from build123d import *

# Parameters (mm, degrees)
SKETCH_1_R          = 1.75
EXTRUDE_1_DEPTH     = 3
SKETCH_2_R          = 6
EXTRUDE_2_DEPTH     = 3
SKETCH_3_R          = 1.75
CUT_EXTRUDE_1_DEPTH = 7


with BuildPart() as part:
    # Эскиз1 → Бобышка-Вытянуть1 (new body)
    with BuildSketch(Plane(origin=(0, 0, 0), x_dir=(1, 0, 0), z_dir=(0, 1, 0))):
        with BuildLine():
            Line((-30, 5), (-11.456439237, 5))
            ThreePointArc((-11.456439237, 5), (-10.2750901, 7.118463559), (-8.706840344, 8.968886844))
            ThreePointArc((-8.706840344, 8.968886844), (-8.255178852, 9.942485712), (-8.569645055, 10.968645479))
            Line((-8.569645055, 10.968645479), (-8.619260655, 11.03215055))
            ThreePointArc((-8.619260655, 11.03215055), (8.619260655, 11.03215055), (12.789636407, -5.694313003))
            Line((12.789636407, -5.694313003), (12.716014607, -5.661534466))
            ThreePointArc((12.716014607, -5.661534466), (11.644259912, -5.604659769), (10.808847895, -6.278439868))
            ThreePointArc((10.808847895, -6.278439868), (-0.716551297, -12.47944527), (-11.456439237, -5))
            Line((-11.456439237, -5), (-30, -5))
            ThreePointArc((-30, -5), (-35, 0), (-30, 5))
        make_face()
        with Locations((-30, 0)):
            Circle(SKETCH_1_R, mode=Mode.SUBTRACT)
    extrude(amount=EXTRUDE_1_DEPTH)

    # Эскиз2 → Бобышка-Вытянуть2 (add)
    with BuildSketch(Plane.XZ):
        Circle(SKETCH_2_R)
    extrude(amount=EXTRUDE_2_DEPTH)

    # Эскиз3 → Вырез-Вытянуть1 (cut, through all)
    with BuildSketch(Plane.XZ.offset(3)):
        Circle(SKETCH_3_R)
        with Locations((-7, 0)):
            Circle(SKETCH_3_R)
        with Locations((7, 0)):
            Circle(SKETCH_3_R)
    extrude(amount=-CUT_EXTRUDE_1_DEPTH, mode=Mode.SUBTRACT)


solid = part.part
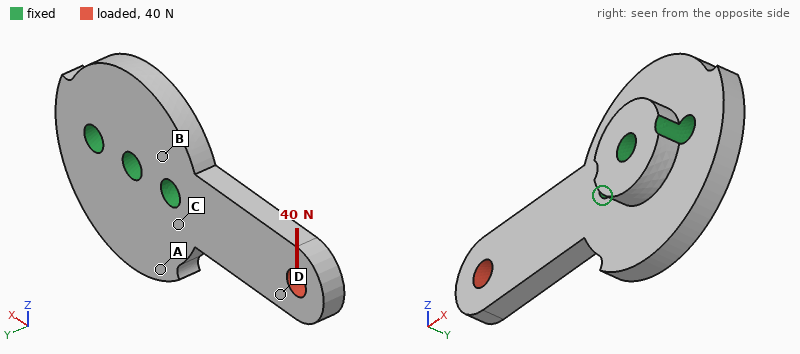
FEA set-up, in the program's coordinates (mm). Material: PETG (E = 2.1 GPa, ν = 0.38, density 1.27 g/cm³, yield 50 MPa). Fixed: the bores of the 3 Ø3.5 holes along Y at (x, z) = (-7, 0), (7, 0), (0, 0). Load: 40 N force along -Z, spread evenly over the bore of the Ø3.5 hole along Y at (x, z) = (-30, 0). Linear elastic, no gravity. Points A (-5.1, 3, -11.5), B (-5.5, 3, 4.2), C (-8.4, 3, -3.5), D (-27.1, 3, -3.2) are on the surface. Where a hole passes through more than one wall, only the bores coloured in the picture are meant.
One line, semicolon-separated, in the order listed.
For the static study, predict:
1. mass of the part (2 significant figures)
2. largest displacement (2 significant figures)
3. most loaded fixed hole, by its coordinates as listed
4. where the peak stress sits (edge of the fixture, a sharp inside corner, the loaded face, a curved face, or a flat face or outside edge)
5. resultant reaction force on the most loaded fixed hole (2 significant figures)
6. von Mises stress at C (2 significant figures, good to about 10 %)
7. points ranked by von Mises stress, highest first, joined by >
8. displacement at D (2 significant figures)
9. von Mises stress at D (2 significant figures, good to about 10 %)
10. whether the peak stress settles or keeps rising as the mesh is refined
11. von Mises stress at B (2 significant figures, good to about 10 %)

3.1 g; 0.43 mm; (-7, 0); a sharp inside corner; 80 N; 6.4 MPa; C > B > D > A; 0.27 mm; 2.2 MPa; keeps rising; 4.3 MPa
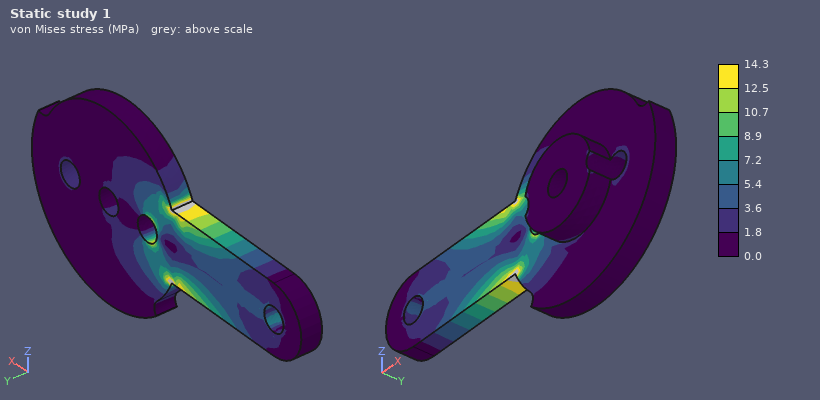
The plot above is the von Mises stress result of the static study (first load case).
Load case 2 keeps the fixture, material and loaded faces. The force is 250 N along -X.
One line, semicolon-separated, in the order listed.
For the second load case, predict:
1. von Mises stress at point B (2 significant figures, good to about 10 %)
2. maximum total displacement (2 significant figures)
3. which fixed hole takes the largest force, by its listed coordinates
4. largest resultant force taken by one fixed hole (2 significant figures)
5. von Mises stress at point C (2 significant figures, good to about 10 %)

2.8 MPa; 0.12 mm; (-7, 0); 200 N; 4.3 MPa
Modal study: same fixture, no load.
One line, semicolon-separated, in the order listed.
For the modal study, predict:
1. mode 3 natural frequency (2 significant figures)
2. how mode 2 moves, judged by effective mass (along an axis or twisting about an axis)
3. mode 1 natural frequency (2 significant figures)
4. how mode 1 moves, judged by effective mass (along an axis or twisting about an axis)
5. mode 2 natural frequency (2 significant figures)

4300 Hz; along Z; 1000 Hz; along Y; 2800 Hz
